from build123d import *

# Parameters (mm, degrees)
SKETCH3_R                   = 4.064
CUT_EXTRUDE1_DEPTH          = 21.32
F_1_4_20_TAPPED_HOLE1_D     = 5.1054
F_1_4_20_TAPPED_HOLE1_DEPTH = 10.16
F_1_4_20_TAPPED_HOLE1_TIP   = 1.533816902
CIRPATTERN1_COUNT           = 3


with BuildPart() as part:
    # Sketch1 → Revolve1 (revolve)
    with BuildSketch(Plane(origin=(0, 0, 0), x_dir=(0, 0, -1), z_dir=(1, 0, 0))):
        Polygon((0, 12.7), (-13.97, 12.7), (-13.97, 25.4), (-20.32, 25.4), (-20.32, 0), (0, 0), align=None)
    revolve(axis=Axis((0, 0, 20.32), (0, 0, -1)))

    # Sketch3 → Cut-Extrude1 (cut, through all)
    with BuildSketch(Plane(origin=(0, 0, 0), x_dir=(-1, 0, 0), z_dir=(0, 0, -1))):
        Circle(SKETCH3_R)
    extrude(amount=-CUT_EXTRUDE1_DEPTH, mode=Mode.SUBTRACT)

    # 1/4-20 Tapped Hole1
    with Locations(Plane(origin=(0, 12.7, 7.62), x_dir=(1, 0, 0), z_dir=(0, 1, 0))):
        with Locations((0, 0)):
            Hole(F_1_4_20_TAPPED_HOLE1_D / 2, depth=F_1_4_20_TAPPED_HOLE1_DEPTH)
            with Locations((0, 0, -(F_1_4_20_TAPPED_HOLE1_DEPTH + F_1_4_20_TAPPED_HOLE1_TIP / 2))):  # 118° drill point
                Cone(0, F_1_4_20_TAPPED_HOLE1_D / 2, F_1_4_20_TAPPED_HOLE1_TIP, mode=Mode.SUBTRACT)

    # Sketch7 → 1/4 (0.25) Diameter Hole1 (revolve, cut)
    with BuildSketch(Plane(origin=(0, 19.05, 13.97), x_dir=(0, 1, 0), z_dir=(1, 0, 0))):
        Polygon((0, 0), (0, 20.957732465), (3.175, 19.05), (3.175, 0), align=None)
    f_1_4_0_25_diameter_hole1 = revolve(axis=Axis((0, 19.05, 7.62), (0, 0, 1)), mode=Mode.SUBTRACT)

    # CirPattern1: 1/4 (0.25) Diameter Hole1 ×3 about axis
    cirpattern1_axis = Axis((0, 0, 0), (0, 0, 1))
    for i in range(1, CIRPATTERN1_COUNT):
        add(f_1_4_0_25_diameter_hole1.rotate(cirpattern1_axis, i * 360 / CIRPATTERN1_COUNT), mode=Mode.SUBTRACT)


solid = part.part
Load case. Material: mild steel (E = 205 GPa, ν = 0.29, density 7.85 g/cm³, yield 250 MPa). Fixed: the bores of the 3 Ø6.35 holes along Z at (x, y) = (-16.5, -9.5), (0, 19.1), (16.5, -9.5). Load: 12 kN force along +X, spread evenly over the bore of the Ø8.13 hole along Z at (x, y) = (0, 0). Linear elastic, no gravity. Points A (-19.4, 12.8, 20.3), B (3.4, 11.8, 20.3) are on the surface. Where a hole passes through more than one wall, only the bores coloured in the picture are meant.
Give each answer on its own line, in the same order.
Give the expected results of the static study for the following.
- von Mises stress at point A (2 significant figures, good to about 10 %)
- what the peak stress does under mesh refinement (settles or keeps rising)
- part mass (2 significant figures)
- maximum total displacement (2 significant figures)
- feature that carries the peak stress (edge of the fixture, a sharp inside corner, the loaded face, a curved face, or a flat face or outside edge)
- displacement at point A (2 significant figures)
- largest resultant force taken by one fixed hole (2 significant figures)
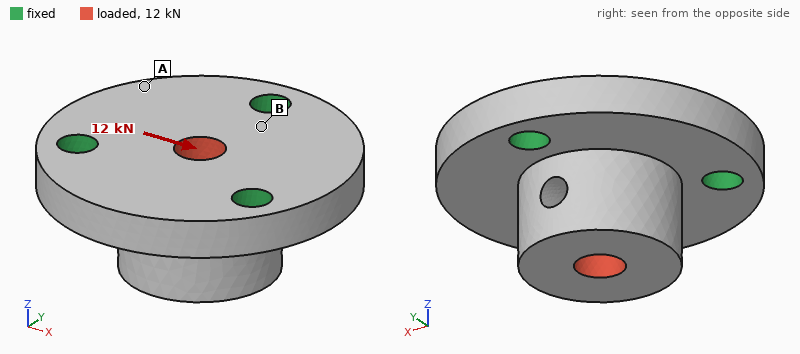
32 MPa
keeps rising
140 g
11 µm
edge of the fixture
4.3 µm
5.2 kN
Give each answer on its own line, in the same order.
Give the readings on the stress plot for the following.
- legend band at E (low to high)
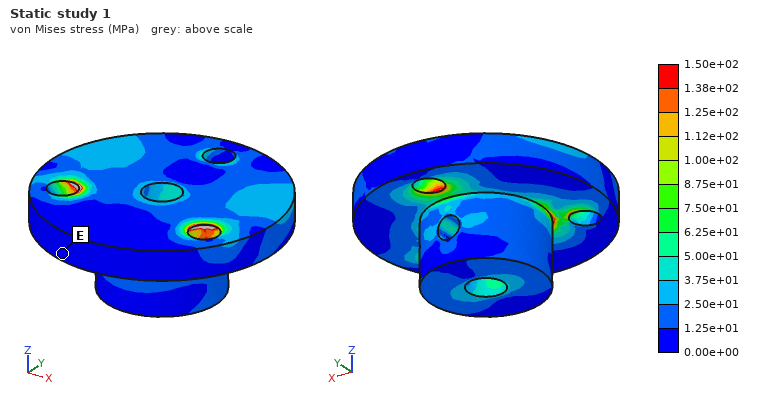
0.00e+00 to 1.25e+01 MPa
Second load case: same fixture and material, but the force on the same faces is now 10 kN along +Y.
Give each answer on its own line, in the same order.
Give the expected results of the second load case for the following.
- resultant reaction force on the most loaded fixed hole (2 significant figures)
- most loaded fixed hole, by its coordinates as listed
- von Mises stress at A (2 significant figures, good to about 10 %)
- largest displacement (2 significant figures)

4.7 kN
(0, 19.1)
19 MPa
9.9 µm
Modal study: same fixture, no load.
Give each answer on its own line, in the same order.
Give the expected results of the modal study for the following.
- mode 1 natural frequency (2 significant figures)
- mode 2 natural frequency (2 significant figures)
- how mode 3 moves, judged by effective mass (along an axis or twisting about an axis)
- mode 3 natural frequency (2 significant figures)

18 kHz
18 kHz
along Z
21 kHz
